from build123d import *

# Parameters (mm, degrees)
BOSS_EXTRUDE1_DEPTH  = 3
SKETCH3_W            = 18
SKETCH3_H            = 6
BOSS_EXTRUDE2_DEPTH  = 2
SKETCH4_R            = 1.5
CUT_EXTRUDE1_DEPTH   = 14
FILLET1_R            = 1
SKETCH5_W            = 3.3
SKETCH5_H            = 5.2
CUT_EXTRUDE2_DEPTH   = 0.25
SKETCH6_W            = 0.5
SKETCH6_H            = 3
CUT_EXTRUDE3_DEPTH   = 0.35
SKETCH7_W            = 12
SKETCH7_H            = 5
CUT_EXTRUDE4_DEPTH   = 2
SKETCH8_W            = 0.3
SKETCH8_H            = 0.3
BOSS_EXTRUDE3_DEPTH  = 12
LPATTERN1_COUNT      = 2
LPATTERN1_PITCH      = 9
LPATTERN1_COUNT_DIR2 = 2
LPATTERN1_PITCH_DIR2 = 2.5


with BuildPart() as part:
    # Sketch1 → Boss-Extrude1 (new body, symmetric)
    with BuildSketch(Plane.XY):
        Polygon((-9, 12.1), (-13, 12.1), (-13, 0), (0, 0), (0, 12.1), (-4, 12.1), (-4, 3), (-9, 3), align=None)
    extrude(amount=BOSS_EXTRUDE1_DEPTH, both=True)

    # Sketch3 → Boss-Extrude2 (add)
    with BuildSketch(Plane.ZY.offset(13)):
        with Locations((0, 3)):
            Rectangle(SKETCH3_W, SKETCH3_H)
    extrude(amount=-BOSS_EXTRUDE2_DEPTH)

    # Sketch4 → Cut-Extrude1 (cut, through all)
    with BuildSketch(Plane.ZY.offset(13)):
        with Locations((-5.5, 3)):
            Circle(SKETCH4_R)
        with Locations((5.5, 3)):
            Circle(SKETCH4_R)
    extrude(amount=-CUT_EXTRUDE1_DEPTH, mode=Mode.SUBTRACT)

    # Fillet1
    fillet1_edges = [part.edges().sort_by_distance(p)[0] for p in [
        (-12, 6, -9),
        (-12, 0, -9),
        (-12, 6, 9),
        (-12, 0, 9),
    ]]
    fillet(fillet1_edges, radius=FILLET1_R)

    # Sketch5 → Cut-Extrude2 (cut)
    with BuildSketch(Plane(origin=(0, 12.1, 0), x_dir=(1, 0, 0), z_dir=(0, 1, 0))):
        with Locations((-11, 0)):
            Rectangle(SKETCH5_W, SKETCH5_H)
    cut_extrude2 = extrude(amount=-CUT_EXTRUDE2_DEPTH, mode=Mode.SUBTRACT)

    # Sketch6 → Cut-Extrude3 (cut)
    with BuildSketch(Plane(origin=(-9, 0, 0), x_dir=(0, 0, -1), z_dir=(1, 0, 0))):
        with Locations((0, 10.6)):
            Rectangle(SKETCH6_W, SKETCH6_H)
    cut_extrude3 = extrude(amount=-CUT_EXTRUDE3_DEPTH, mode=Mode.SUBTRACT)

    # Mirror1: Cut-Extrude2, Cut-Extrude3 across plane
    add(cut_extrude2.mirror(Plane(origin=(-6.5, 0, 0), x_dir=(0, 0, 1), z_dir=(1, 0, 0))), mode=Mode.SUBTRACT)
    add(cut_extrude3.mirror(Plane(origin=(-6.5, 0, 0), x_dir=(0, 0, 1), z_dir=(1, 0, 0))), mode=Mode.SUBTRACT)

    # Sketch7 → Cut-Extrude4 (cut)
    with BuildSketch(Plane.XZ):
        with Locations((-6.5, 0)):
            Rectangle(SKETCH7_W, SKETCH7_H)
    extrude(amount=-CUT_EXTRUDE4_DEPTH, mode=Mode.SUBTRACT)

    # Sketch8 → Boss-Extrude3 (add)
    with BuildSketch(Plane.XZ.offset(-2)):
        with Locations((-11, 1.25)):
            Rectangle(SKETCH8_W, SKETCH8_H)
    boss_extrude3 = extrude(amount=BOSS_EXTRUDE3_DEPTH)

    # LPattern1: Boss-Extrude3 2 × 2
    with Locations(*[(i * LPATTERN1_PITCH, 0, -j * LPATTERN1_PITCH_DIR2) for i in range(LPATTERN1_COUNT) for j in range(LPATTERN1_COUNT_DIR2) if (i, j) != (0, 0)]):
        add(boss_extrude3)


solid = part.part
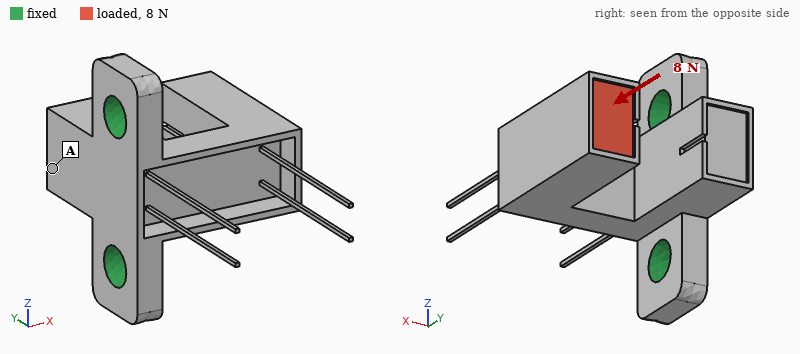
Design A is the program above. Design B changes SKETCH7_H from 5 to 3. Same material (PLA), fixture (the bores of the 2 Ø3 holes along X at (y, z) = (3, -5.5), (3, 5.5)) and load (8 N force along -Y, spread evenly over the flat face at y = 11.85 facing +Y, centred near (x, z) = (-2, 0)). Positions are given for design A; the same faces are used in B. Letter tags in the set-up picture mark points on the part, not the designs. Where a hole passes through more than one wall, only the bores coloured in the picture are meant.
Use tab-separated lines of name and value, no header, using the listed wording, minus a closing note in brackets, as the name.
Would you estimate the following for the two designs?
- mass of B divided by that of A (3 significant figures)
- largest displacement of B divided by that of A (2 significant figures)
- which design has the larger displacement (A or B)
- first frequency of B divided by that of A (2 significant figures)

mass of B divided by that of A	1.07
largest displacement of B divided by that of A	0.57
which design has the larger displacement	A
first frequency of B divided by that of A	1.00
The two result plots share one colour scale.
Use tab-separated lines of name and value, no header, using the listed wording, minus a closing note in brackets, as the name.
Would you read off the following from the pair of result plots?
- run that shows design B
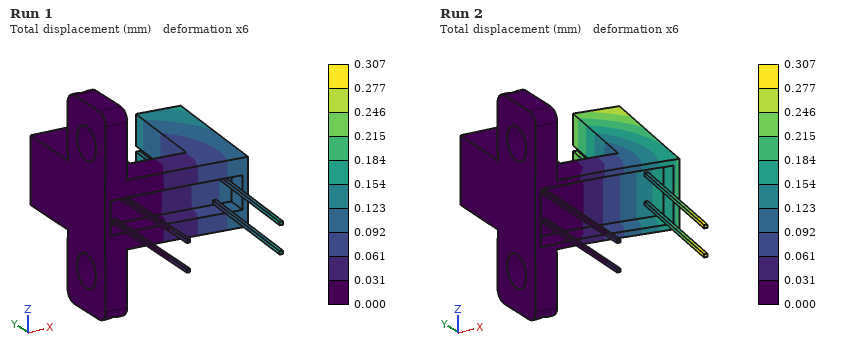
run that shows design B	Run 1
